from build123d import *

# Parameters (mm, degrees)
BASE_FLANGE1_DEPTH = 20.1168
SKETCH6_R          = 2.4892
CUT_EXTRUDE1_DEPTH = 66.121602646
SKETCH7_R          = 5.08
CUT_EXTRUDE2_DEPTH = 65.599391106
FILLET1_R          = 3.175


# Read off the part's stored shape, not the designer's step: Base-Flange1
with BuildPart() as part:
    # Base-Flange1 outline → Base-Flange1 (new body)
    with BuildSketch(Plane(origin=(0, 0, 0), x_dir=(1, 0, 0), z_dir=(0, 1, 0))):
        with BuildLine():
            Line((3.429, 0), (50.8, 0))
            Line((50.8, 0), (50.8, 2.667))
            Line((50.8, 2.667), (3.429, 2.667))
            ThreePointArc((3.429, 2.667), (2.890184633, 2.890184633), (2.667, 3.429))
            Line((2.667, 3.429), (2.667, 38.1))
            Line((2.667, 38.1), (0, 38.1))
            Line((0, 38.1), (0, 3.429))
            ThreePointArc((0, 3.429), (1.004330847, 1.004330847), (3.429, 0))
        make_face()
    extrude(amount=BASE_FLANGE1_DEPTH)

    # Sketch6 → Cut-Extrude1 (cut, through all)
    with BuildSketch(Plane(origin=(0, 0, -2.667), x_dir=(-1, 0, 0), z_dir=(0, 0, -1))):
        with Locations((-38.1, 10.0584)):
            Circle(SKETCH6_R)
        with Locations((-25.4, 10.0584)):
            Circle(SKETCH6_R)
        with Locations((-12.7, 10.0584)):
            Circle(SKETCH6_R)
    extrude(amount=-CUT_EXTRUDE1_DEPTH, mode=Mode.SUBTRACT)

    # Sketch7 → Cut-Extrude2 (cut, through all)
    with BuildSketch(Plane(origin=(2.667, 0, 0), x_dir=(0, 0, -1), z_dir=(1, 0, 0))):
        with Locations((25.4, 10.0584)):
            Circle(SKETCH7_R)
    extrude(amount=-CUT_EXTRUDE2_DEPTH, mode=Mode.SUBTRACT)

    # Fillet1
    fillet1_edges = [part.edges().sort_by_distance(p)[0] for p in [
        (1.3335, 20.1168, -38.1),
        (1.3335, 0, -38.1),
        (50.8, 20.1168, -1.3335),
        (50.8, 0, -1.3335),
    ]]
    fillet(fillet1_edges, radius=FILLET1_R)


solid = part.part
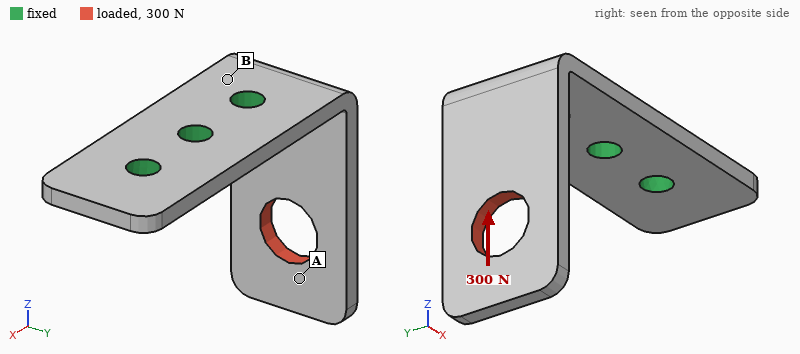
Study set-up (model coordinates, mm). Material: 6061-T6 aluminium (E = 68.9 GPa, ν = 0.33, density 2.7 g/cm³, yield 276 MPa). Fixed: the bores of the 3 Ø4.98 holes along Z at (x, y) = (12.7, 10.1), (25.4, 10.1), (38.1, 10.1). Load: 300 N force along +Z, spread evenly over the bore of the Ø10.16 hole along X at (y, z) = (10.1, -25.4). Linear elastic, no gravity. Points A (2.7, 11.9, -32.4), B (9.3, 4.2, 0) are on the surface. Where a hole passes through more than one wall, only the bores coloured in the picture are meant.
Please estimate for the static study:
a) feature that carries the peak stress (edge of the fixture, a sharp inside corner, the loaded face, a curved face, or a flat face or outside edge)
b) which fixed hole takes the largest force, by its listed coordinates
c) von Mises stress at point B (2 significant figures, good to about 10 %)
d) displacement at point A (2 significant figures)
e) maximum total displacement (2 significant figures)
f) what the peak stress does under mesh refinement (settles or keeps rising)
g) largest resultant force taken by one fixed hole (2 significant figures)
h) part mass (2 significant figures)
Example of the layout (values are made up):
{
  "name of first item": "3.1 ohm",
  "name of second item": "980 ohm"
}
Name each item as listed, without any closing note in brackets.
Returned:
{
  "feature that carries the peak stress": "edge of the fixture",
  "which fixed hole takes the largest force, by its listed coordinates": "(12.7, 10.1)",
  "von Mises stress at point B": "68 MPa",
  "displacement at point A": "0.23 mm",
  "maximum total displacement": "0.27 mm",
  "what the peak stress does under mesh refinement": "keeps rising",
  "largest resultant force taken by one fixed hole": "350 N",
  "part mass": "11 g"
}
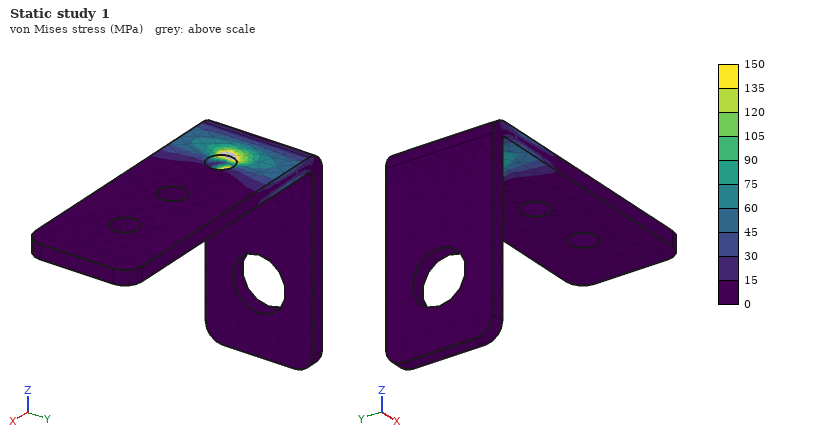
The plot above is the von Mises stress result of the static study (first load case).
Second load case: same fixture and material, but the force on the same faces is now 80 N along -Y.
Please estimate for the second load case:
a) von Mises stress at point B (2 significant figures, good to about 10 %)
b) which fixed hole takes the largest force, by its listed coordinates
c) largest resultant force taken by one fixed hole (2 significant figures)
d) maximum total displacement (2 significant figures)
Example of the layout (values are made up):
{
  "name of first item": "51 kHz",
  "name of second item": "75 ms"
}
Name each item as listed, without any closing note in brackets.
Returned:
{
  "von Mises stress at point B": "38 MPa",
  "which fixed hole takes the largest force, by its listed coordinates": "(12.7, 10.1)",
  "largest resultant force taken by one fixed hole": "110 N",
  "maximum total displacement": "0.18 mm"
}
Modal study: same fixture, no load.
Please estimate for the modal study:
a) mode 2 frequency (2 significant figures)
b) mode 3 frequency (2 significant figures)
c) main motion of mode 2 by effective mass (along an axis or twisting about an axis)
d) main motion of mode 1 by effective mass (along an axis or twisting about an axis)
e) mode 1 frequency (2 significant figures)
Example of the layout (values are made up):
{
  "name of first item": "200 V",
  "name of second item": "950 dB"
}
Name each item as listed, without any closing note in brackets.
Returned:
{
  "mode 2 frequency": "2100 Hz",
  "mode 3 frequency": "5600 Hz",
  "main motion of mode 2 by effective mass": "along Y",
  "main motion of mode 1 by effective mass": "along X",
  "mode 1 frequency": "1200 Hz"
}
